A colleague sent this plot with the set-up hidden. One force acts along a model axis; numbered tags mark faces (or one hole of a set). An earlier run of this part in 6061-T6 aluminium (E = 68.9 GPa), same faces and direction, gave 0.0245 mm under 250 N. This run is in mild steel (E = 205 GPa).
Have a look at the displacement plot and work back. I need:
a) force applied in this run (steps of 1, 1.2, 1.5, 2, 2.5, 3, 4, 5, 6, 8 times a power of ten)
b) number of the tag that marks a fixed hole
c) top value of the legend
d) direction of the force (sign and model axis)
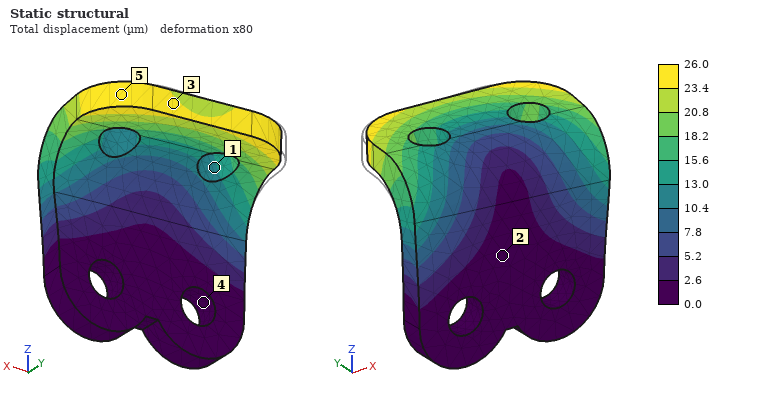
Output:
800 N
4
26.0 µm
+X
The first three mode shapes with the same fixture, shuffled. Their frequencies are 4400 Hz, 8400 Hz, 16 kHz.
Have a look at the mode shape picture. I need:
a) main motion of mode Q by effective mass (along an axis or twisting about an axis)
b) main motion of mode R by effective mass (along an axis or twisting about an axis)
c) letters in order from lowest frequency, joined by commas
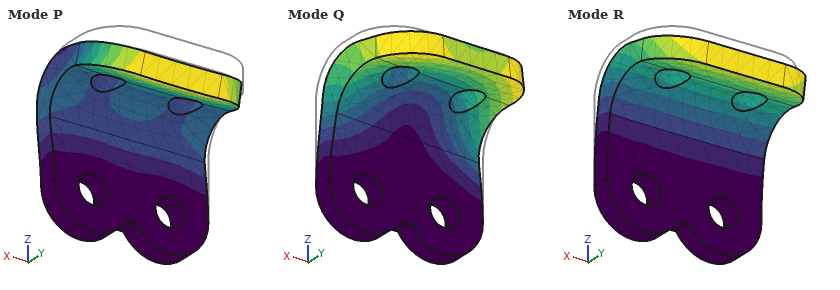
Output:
along X
along Y
R, Q, P
